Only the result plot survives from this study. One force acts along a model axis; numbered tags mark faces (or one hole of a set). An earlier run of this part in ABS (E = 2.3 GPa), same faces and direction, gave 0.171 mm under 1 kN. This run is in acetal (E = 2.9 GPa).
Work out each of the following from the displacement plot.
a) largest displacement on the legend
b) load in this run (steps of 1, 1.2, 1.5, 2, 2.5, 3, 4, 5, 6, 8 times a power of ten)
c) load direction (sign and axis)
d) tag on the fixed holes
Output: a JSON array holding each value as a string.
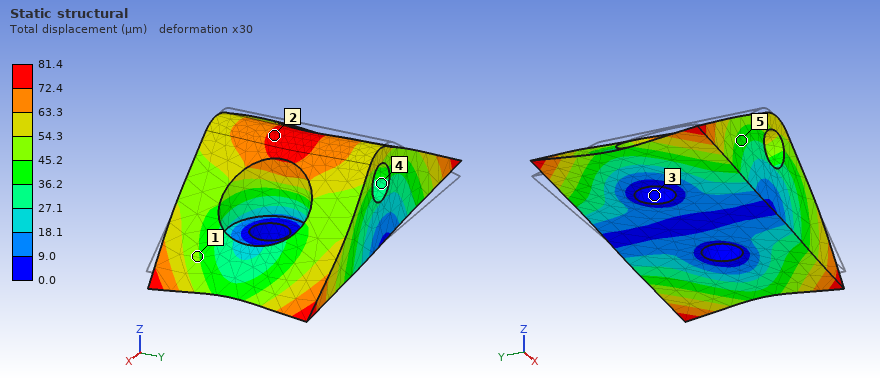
["81.4 µm", "600 N", "+X", "3"]
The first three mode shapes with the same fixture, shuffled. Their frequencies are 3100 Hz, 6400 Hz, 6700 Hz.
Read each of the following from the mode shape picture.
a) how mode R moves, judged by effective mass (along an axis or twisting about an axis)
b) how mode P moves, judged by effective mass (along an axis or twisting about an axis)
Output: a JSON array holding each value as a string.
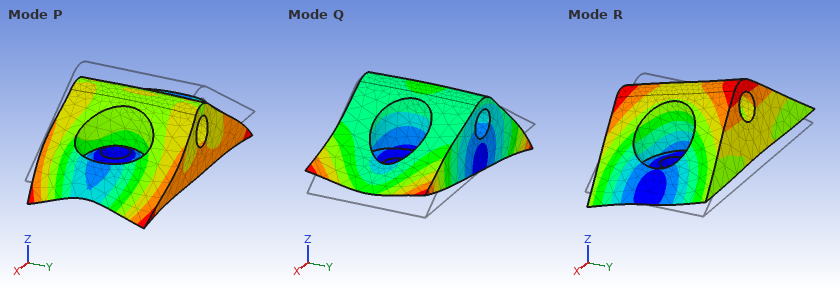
["along Y", "along Z"]
